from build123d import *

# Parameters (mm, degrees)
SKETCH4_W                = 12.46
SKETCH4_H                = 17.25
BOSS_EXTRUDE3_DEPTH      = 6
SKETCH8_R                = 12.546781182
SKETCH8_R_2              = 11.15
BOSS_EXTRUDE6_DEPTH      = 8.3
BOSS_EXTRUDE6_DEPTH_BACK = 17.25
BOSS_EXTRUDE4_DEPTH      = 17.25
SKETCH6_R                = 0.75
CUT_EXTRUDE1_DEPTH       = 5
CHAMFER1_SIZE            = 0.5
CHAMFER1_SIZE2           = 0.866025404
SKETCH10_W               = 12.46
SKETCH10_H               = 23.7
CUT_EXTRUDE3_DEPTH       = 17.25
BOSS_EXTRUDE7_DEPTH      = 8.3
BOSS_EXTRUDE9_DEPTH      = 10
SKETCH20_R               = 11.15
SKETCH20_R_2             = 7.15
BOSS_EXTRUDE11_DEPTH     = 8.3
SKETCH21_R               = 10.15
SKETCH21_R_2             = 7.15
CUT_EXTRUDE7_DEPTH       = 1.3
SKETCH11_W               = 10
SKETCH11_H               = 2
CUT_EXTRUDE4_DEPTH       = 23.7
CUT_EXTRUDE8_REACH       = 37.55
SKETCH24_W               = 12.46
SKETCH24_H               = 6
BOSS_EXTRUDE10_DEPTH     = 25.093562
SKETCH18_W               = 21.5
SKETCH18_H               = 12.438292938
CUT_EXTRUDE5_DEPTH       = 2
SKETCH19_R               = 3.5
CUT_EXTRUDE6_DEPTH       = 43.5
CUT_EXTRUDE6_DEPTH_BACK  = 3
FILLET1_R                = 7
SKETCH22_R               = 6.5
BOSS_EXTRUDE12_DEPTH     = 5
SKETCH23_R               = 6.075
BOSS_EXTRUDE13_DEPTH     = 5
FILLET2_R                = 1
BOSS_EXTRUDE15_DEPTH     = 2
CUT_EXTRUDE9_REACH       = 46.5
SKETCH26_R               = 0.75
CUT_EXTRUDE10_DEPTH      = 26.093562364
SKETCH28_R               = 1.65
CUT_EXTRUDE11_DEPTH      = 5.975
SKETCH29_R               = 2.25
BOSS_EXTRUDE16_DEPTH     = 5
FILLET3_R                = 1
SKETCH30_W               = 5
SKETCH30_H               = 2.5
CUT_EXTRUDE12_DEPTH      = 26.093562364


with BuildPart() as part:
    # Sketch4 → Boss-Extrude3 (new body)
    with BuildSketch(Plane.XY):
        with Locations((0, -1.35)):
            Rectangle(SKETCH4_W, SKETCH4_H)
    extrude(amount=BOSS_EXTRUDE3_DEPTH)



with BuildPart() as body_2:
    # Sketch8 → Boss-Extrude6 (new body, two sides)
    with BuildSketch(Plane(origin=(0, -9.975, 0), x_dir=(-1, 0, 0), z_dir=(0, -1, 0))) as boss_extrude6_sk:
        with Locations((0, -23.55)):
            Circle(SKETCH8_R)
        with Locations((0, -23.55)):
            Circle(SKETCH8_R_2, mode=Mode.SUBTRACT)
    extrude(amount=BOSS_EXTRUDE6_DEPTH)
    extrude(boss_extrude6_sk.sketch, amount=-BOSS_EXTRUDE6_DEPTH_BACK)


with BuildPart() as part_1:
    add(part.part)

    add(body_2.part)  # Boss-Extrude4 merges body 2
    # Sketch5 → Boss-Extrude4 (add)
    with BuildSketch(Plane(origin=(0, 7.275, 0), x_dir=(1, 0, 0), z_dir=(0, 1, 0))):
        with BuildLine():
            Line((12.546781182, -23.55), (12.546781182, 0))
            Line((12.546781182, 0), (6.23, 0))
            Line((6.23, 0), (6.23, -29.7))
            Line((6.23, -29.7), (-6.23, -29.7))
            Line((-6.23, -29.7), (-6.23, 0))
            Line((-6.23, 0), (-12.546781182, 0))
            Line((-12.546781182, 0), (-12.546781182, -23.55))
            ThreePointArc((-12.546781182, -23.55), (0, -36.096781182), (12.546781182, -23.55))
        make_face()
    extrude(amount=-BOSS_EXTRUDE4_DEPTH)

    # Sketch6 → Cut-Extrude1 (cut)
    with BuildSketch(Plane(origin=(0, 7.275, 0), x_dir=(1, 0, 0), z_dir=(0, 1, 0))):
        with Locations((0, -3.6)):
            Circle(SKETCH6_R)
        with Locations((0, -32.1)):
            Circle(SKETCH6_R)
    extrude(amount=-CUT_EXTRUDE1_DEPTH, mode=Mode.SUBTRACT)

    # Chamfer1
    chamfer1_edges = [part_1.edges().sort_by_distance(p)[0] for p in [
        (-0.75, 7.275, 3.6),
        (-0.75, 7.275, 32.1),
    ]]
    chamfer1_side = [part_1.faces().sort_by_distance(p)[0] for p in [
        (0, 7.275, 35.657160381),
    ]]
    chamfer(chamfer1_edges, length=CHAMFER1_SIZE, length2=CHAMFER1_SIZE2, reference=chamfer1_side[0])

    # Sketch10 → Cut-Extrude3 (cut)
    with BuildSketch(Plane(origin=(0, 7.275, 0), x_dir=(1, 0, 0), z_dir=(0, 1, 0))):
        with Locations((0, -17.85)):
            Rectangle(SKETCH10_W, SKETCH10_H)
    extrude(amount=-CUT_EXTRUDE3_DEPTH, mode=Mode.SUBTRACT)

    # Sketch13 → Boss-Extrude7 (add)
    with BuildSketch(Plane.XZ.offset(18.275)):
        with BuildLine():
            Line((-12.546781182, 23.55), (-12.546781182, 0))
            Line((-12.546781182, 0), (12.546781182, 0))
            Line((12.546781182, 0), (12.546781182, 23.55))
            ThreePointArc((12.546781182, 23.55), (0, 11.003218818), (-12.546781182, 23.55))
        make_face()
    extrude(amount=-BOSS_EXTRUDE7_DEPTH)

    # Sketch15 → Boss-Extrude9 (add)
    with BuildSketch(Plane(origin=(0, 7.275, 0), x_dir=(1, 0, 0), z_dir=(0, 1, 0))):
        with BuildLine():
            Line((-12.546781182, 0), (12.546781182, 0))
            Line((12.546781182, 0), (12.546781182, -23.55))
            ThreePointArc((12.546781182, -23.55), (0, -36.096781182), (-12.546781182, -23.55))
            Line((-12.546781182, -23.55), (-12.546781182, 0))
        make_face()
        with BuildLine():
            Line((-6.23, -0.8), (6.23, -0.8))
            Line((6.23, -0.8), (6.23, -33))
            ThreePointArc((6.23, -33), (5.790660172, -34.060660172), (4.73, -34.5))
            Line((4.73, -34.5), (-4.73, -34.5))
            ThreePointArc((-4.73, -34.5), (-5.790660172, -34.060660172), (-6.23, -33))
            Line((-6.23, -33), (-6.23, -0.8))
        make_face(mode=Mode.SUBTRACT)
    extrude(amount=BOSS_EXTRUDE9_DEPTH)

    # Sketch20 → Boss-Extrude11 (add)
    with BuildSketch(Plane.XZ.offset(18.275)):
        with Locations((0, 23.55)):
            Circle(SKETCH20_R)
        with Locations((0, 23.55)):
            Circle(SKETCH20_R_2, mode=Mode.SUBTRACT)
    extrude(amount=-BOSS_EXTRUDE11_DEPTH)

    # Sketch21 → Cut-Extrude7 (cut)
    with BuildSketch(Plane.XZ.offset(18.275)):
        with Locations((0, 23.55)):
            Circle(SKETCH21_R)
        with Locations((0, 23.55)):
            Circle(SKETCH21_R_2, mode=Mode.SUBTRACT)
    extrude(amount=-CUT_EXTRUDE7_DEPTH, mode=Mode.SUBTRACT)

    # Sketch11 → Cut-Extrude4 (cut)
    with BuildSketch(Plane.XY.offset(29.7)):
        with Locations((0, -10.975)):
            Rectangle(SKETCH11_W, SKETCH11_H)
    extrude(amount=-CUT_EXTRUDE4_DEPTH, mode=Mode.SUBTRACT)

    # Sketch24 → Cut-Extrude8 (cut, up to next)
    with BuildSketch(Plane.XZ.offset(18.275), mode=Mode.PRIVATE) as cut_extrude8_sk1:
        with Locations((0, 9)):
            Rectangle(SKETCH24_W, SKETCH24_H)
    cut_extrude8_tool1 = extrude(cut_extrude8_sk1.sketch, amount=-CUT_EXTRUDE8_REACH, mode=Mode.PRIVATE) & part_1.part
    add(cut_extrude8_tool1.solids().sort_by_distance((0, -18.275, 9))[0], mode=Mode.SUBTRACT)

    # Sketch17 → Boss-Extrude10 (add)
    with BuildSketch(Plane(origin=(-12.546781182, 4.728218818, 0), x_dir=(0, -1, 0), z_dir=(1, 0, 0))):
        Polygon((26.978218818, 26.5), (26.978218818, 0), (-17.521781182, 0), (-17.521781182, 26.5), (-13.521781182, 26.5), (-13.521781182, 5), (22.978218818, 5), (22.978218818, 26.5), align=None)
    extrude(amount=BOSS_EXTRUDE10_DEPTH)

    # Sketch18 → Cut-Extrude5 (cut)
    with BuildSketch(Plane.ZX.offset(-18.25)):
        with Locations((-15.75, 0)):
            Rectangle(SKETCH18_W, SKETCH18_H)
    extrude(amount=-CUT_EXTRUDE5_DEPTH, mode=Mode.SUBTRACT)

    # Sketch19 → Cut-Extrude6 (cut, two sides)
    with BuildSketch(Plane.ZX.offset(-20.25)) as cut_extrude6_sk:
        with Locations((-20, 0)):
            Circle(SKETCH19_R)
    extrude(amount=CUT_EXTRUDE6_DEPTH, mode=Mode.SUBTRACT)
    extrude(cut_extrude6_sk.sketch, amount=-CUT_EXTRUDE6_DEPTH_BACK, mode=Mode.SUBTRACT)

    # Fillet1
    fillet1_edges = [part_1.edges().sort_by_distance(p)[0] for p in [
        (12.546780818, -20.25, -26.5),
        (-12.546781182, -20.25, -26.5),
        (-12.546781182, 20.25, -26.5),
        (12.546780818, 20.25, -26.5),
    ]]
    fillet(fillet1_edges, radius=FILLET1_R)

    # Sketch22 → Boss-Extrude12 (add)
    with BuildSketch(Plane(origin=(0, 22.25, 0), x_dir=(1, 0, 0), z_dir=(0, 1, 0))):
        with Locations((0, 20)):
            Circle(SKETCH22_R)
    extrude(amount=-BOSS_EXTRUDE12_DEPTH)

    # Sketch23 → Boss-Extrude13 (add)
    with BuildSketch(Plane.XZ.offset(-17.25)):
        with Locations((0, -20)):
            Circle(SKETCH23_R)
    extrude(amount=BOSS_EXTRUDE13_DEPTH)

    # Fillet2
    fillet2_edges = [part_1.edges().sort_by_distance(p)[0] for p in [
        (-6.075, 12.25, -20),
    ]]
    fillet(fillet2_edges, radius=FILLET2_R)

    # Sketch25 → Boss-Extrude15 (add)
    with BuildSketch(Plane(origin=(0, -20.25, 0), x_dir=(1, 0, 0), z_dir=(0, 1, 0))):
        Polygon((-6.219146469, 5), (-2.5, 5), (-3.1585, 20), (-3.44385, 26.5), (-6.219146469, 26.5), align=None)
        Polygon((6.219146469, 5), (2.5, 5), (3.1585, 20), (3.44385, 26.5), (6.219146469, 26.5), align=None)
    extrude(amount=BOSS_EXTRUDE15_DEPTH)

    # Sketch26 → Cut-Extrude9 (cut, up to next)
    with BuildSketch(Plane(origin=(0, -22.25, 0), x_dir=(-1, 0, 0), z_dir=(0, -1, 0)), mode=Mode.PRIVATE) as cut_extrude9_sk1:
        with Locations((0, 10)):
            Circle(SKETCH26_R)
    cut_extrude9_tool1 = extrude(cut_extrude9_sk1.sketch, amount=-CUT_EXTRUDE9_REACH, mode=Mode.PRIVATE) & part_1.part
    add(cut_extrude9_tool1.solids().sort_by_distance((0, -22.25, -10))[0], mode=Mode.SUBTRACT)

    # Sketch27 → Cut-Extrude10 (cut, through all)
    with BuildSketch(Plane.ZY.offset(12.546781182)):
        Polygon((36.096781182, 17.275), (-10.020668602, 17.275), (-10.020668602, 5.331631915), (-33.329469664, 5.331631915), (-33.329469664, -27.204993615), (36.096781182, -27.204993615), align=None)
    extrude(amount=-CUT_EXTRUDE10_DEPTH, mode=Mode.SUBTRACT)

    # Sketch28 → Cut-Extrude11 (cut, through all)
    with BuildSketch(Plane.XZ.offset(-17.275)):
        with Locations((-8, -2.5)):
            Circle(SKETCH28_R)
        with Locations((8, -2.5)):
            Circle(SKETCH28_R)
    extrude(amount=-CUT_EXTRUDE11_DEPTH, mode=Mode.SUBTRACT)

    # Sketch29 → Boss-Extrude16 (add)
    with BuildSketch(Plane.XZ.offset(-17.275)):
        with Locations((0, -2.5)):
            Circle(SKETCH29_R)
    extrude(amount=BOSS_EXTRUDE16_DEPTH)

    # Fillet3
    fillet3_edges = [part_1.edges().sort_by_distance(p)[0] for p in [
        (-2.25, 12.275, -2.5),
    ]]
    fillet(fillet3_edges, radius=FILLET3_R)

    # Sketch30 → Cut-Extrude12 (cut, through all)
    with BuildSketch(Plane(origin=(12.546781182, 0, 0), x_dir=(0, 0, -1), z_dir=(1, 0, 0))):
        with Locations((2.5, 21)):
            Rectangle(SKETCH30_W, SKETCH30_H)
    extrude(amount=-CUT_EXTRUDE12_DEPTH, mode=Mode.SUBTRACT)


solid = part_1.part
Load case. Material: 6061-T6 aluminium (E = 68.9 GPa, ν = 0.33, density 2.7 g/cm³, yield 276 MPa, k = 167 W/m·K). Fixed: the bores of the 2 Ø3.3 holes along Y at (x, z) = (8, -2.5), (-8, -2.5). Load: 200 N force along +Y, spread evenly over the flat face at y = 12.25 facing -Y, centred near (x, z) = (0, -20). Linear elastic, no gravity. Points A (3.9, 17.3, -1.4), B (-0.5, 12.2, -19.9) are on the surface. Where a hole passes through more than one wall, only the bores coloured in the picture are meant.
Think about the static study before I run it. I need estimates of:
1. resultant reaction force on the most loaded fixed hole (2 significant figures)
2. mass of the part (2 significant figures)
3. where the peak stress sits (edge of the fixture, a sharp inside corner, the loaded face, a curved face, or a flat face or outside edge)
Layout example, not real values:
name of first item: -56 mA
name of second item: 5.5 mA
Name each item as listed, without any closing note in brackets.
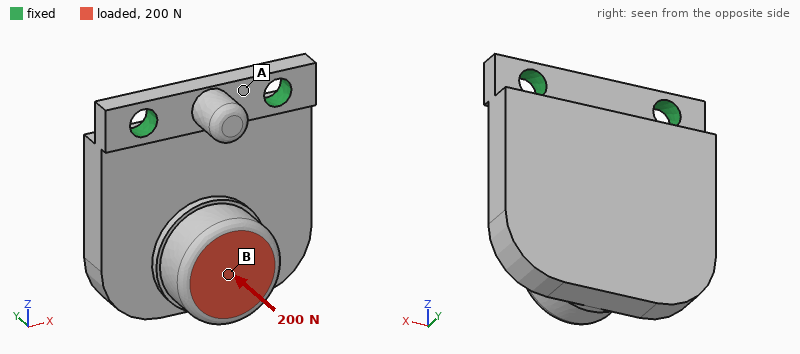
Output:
resultant reaction force on the most loaded fixed hole: 110 N
mass of the part: 8.4 g
where the peak stress sits: a flat face or outside edge
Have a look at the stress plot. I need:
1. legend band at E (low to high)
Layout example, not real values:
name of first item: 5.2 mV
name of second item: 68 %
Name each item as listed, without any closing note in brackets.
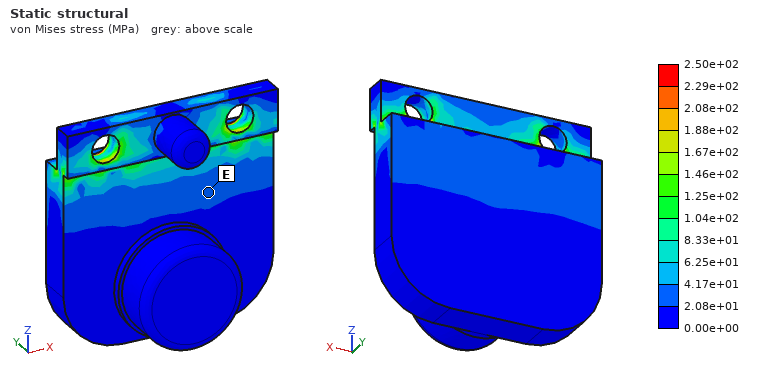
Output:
legend band at E: 2.08e+01 to 4.17e+01 MPa
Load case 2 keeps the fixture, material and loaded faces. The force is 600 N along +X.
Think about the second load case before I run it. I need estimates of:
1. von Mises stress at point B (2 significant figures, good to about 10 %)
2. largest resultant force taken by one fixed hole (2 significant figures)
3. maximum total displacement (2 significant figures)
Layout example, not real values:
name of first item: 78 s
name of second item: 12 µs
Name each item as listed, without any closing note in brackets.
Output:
von Mises stress at point B: 17 MPa
largest resultant force taken by one fixed hole: 670 N
maximum total displacement: 64 µm
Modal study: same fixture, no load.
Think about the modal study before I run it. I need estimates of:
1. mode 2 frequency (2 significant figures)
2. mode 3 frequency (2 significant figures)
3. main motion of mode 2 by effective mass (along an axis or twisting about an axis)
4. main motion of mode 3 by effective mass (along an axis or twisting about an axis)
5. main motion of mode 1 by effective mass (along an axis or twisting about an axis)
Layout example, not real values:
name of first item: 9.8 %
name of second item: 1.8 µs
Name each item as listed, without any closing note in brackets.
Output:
mode 2 frequency: 9700 Hz
mode 3 frequency: 17 kHz
main motion of mode 2 by effective mass: along X
main motion of mode 3 by effective mass: along X
main motion of mode 1 by effective mass: along Y
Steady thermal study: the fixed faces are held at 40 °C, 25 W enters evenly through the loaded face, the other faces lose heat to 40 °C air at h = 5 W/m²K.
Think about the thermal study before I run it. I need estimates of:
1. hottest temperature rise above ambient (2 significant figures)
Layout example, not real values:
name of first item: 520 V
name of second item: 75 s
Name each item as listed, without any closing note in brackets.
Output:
hottest temperature rise above ambient: 41 K
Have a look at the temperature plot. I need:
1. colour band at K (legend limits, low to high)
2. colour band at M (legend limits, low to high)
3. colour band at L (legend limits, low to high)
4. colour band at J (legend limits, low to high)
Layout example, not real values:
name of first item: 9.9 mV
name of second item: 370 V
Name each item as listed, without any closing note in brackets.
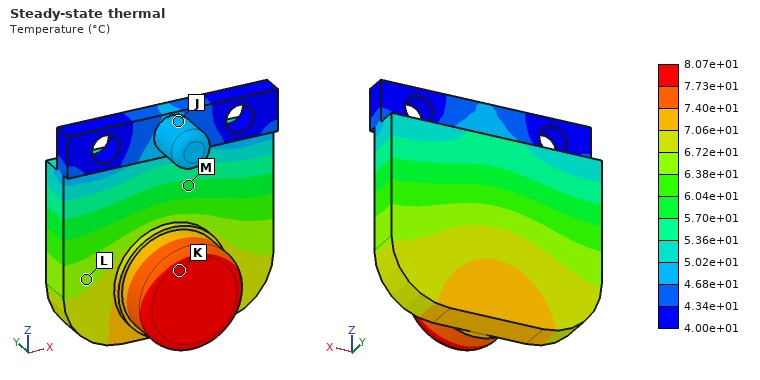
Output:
colour band at K: 7.73e+01 to 8.07e+01 °C
colour band at M: 5.70e+01 to 6.04e+01 °C
colour band at L: 6.38e+01 to 6.72e+01 °C
colour band at J: 4.68e+01 to 5.02e+01 °C
